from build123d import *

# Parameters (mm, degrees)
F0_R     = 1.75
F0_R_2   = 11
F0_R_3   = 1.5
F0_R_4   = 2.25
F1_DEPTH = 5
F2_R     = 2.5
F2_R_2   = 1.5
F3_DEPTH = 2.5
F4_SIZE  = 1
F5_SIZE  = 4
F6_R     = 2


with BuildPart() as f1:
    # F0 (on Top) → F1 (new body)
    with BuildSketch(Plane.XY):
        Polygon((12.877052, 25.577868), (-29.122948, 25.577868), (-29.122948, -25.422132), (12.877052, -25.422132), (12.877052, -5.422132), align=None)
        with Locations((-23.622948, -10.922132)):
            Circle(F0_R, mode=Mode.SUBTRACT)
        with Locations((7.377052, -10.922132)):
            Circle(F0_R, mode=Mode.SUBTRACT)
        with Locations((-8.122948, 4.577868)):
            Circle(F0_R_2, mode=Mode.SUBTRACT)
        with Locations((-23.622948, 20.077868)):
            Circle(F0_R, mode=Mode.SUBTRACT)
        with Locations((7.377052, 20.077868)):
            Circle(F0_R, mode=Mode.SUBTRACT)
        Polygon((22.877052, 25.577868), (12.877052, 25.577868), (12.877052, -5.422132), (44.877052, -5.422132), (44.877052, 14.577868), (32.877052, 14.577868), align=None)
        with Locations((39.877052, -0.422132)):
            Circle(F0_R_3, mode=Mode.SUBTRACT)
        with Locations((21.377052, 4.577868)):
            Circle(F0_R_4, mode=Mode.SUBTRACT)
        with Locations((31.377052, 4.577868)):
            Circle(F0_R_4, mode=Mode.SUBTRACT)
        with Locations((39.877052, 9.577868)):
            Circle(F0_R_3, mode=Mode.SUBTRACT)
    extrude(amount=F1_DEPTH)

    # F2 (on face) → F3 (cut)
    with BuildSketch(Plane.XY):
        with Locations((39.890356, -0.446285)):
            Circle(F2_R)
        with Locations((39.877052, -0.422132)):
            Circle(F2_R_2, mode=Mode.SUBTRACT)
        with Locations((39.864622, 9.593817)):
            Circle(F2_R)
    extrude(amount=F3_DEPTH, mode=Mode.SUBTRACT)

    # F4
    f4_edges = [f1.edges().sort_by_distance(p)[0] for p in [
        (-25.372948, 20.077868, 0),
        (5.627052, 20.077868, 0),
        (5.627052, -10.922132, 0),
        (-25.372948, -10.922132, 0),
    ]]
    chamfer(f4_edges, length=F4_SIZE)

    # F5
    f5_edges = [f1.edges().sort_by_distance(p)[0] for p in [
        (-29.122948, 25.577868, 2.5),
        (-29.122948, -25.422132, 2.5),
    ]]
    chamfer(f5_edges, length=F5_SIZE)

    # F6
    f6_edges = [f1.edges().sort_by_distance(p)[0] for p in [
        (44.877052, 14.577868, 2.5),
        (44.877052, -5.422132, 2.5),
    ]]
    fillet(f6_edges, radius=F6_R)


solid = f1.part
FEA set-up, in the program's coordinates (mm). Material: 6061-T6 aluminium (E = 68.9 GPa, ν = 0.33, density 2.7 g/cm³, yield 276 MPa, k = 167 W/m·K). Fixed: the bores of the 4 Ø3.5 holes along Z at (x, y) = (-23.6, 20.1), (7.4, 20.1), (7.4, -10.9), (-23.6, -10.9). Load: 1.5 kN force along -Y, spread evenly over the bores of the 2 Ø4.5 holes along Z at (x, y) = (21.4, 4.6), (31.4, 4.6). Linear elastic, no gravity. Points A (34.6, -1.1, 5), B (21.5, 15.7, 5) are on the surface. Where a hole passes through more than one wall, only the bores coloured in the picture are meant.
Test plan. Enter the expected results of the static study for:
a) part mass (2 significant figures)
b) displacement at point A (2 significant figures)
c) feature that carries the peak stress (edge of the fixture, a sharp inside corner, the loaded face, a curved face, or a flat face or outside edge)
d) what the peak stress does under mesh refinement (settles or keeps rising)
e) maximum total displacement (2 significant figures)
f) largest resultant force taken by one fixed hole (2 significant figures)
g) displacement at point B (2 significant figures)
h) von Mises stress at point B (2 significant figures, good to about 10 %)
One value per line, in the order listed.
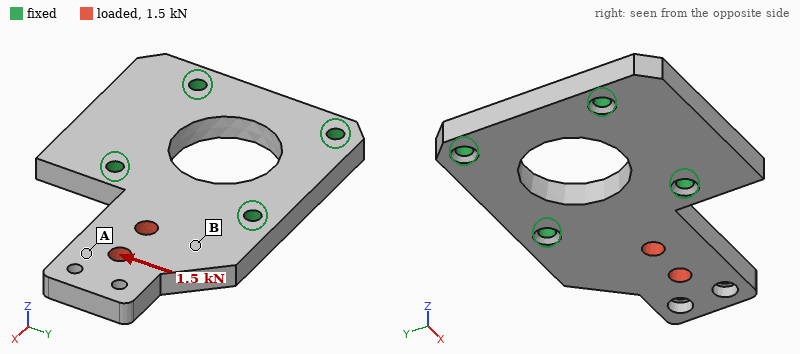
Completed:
33 g
21 µm
edge of the fixture
keeps rising
25 µm
1.2 kN
9.9 µm
17 MPa
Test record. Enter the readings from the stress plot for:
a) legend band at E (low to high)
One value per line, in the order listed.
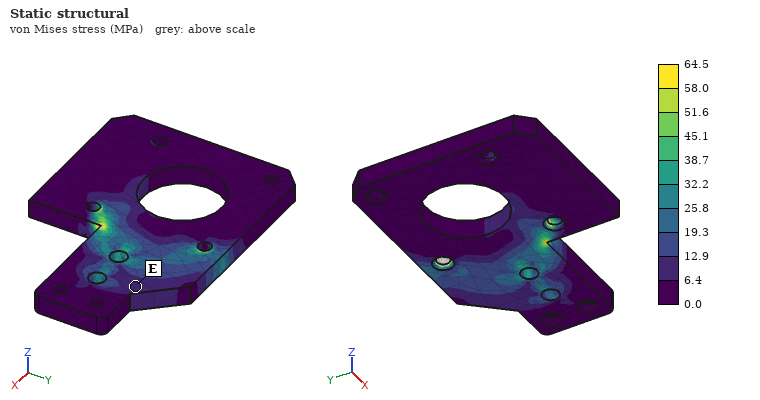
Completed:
6.4 to 12.9 MPa
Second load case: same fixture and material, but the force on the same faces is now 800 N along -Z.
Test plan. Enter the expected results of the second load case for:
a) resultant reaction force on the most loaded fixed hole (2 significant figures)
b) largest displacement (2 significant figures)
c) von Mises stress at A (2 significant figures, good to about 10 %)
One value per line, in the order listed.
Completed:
510 N
0.36 mm
23 MPa
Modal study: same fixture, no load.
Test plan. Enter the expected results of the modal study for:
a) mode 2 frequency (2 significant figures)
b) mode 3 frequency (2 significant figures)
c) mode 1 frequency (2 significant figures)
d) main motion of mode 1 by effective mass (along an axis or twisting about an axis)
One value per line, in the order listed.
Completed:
11 kHz
13 kHz
3000 Hz
along Z
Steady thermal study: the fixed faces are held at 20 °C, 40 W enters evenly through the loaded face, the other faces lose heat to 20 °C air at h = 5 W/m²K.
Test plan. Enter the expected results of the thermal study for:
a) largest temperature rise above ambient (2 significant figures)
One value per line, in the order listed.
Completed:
47 K
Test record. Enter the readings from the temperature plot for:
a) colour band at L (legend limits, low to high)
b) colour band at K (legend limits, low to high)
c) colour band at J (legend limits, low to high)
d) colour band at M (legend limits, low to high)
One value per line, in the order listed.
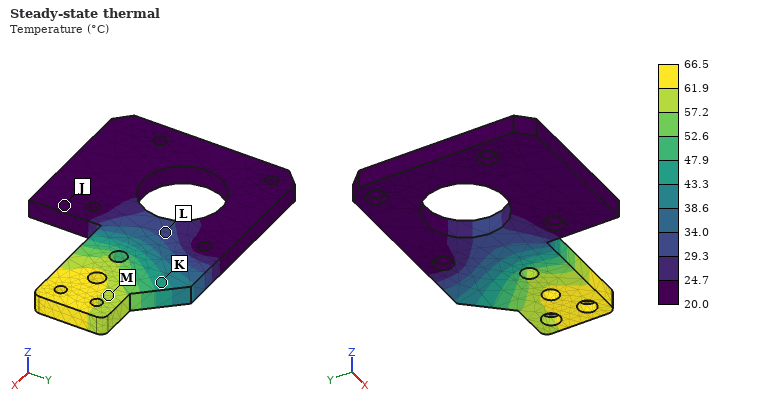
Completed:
29.3 to 34.0 °C
43.3 to 47.9 °C
20.0 to 24.7 °C
57.2 to 61.9 °C
